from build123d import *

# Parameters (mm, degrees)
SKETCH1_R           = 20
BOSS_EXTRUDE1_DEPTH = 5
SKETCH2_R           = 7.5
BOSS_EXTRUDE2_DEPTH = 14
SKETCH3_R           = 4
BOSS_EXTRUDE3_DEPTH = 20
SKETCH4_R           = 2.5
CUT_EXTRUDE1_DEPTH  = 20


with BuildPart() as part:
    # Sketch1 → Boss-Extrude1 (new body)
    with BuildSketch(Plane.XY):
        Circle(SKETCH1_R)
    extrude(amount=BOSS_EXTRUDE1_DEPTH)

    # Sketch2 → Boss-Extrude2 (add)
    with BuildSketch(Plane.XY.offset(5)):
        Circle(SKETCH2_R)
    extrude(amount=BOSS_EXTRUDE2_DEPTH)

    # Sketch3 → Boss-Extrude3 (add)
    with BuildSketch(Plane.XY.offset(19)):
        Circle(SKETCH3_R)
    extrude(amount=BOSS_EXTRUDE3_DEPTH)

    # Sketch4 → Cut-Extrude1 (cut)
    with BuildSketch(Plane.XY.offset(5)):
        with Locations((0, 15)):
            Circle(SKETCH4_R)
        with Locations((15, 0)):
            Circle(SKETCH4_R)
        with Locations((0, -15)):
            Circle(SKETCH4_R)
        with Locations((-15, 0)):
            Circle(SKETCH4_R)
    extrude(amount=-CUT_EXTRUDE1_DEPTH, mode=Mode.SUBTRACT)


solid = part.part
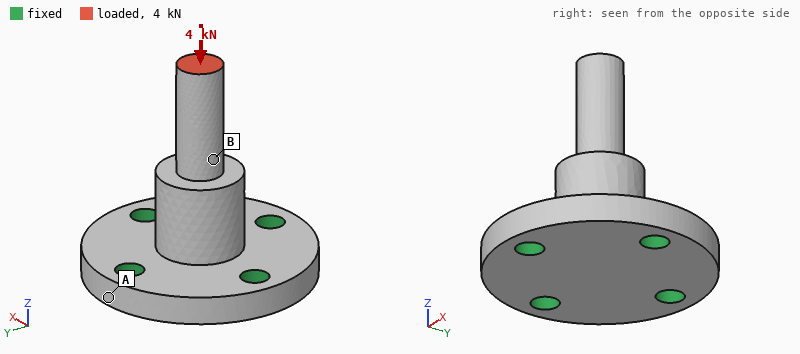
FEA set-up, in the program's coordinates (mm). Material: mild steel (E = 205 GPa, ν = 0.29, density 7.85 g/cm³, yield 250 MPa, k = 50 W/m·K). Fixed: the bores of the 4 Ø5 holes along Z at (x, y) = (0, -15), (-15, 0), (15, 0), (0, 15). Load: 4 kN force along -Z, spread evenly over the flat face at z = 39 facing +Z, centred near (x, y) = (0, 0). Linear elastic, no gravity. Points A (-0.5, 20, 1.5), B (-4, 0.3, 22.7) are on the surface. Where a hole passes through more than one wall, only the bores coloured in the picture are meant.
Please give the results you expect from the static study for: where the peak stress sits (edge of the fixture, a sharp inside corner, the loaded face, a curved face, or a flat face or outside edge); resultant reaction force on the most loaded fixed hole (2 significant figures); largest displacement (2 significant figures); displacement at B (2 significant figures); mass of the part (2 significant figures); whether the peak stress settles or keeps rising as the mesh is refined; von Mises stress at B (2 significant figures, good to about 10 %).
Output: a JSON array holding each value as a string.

["edge of the fixture", "1.0 kN", "14 µm", "7.2 µm", "74 g", "keeps rising", "77 MPa"]
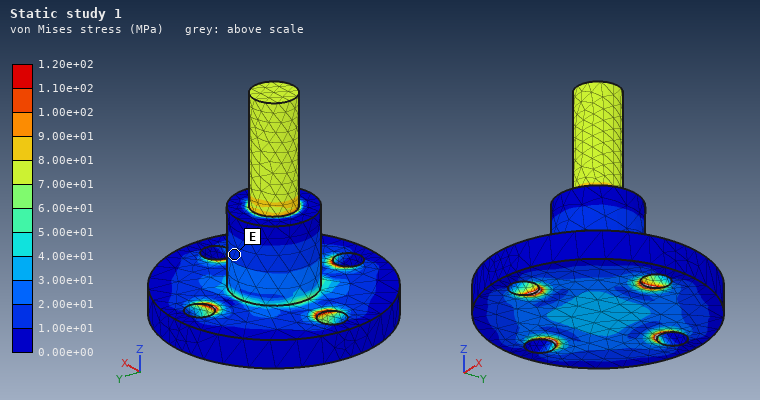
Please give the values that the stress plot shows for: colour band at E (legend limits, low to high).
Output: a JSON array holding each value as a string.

["1.00e+01 to 2.00e+01 MPa"]
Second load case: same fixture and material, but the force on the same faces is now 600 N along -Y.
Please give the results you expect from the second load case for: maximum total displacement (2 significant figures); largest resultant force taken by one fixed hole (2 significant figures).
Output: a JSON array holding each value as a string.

["77 µm", "890 N"]
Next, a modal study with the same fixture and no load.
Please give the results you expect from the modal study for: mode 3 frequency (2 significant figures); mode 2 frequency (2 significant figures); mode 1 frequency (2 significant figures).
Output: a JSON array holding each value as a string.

["23 kHz", "8400 Hz", "8400 Hz"]
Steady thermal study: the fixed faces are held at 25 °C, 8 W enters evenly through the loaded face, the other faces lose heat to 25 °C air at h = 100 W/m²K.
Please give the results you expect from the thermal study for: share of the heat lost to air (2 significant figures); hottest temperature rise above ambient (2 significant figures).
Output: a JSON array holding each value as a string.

["37 %", "69 K"]
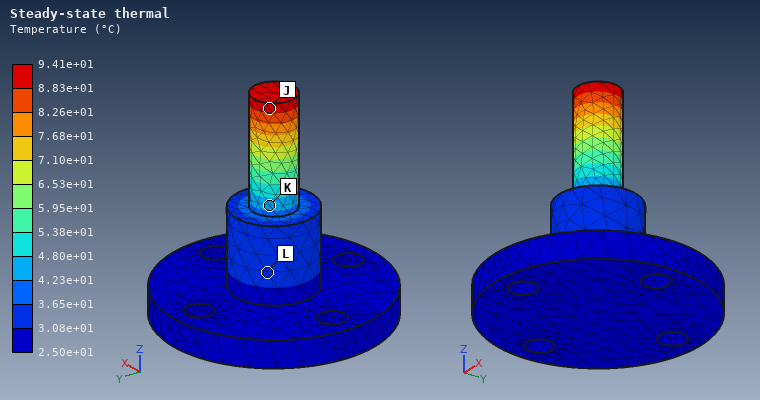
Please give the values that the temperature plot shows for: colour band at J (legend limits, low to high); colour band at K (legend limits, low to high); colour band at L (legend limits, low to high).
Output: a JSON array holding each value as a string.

["8.83e+01 to 9.41e+01 °C", "4.23e+01 to 4.80e+01 °C", "3.08e+01 to 3.65e+01 °C"]
